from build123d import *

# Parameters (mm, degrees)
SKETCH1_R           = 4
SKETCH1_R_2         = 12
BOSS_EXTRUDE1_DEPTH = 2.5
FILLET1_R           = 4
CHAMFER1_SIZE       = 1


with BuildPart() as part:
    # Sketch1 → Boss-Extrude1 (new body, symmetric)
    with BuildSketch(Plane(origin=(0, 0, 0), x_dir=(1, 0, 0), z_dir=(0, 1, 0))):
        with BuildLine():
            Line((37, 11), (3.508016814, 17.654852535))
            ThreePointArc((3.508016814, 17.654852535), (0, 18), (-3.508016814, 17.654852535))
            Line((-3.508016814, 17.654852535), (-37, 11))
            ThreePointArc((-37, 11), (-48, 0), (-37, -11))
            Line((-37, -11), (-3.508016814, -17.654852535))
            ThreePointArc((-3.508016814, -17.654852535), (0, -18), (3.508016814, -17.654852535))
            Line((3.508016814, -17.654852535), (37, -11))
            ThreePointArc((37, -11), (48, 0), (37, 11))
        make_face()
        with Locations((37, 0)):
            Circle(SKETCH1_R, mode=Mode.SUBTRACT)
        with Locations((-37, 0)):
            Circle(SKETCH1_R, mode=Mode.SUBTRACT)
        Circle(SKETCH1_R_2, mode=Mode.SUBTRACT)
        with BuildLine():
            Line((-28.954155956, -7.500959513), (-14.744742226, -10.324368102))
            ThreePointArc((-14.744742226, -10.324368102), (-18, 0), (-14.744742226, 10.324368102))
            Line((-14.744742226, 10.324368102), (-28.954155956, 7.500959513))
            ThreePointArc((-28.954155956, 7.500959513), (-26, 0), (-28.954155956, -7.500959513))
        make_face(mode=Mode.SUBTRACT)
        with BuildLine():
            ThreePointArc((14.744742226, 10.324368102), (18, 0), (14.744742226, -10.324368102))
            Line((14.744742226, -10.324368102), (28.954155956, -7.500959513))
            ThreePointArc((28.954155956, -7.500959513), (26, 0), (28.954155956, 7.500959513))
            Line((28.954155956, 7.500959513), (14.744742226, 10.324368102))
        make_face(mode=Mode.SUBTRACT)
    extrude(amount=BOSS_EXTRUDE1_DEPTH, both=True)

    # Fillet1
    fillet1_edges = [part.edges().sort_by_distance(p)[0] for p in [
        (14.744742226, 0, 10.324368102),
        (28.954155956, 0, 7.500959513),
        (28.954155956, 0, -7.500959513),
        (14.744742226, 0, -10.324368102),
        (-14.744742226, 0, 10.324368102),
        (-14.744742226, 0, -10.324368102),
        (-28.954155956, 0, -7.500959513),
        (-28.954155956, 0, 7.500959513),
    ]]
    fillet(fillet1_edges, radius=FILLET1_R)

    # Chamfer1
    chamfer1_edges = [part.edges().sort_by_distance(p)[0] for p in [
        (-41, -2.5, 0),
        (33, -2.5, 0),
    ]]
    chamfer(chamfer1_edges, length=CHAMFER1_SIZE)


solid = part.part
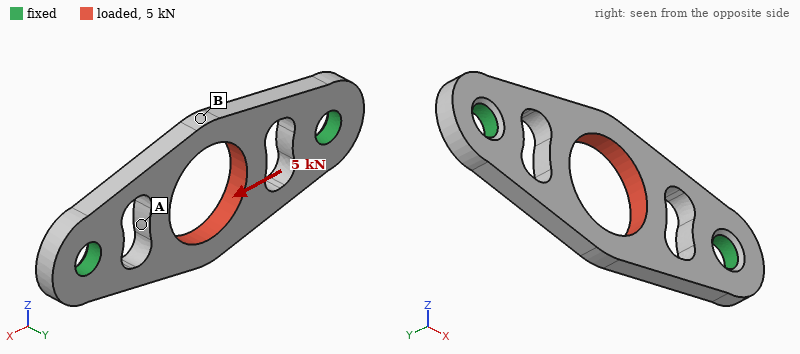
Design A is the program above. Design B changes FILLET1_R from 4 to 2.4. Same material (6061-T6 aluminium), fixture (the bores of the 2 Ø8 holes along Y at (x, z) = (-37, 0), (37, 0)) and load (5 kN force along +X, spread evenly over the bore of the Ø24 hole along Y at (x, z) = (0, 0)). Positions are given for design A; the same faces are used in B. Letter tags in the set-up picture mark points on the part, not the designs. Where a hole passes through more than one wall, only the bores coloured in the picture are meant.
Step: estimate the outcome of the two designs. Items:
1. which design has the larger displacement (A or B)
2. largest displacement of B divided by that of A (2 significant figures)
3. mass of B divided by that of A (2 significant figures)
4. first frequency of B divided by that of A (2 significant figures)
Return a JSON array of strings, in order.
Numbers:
["B", "1.1", "0.98", "0.98"]
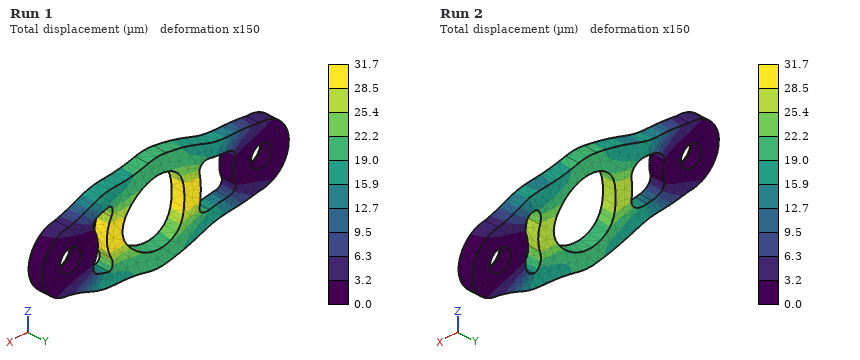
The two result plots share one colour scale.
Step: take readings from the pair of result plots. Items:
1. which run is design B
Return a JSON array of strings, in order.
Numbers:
["Run 1"]
